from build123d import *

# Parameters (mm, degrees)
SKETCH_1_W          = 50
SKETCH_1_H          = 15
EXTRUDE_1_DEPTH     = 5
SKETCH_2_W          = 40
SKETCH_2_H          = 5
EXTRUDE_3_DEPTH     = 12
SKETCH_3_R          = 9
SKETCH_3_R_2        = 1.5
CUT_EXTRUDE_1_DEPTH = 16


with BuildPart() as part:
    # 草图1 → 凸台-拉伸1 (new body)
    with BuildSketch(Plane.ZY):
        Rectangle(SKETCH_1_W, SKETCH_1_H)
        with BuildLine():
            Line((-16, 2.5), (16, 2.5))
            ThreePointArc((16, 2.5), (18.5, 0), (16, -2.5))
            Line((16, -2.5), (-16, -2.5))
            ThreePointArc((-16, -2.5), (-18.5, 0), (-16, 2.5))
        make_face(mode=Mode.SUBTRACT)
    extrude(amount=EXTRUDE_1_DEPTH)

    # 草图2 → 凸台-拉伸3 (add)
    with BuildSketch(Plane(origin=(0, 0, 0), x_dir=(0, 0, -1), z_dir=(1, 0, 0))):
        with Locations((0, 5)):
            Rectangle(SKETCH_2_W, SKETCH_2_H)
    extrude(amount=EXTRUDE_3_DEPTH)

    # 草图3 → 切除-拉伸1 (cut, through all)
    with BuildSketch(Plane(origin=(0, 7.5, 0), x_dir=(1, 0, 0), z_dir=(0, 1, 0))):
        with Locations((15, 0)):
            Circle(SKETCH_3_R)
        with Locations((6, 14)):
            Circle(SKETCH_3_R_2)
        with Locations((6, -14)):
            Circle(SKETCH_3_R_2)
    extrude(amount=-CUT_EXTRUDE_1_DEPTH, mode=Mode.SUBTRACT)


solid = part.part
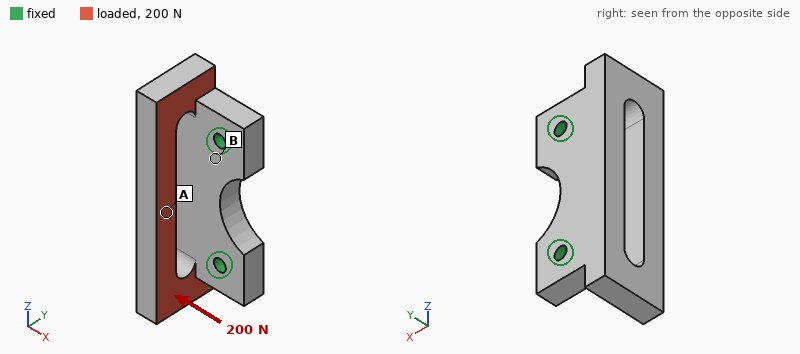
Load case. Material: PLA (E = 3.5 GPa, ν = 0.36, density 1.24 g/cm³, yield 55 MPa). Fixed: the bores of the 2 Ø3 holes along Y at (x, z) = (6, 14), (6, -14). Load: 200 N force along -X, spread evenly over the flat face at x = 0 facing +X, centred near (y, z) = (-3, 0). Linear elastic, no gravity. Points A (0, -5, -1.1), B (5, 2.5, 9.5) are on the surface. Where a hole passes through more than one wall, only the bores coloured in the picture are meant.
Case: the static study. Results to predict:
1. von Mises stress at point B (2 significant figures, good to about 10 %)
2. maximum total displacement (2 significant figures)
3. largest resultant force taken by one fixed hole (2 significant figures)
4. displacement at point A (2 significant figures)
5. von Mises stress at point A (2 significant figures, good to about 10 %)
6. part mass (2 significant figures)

5.0 MPa
0.64 mm
110 N
0.53 mm
13 MPa
6.0 g
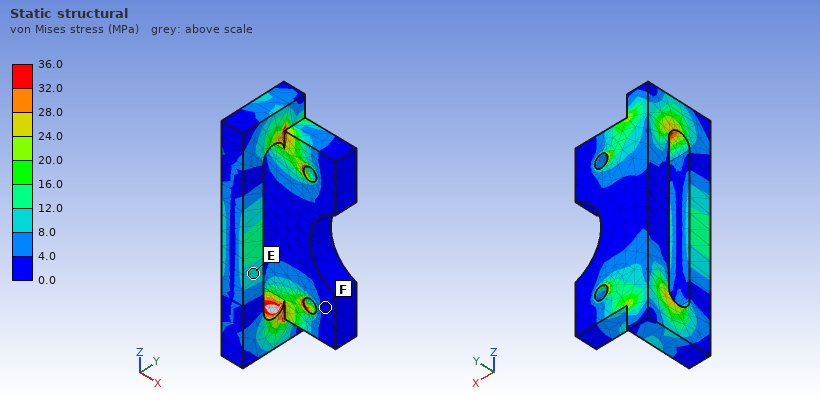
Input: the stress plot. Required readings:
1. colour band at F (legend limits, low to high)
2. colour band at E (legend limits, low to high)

0.0 to 4.0 MPa
8.0 to 12.0 MPa
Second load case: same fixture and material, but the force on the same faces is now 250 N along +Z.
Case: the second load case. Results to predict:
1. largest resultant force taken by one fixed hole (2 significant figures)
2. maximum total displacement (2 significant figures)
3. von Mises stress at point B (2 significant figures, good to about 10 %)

140 N
0.31 mm
3.2 MPa
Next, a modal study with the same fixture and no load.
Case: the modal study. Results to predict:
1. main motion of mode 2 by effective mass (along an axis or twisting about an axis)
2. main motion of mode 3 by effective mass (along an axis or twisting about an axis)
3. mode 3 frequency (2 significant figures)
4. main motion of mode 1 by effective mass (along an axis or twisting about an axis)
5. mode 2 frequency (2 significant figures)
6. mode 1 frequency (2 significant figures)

along Z
along Y
3800 Hz
along X
3200 Hz
2200 Hz
